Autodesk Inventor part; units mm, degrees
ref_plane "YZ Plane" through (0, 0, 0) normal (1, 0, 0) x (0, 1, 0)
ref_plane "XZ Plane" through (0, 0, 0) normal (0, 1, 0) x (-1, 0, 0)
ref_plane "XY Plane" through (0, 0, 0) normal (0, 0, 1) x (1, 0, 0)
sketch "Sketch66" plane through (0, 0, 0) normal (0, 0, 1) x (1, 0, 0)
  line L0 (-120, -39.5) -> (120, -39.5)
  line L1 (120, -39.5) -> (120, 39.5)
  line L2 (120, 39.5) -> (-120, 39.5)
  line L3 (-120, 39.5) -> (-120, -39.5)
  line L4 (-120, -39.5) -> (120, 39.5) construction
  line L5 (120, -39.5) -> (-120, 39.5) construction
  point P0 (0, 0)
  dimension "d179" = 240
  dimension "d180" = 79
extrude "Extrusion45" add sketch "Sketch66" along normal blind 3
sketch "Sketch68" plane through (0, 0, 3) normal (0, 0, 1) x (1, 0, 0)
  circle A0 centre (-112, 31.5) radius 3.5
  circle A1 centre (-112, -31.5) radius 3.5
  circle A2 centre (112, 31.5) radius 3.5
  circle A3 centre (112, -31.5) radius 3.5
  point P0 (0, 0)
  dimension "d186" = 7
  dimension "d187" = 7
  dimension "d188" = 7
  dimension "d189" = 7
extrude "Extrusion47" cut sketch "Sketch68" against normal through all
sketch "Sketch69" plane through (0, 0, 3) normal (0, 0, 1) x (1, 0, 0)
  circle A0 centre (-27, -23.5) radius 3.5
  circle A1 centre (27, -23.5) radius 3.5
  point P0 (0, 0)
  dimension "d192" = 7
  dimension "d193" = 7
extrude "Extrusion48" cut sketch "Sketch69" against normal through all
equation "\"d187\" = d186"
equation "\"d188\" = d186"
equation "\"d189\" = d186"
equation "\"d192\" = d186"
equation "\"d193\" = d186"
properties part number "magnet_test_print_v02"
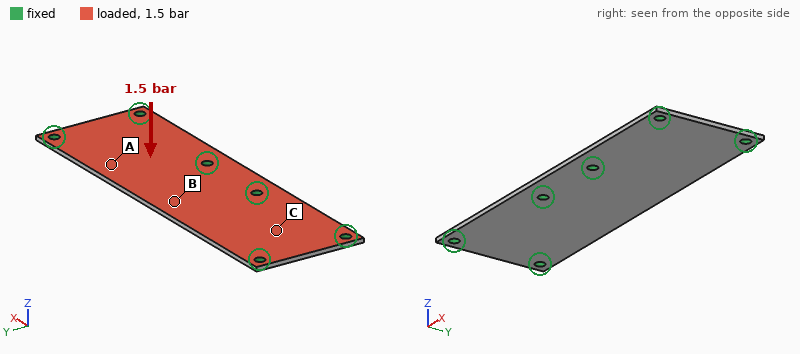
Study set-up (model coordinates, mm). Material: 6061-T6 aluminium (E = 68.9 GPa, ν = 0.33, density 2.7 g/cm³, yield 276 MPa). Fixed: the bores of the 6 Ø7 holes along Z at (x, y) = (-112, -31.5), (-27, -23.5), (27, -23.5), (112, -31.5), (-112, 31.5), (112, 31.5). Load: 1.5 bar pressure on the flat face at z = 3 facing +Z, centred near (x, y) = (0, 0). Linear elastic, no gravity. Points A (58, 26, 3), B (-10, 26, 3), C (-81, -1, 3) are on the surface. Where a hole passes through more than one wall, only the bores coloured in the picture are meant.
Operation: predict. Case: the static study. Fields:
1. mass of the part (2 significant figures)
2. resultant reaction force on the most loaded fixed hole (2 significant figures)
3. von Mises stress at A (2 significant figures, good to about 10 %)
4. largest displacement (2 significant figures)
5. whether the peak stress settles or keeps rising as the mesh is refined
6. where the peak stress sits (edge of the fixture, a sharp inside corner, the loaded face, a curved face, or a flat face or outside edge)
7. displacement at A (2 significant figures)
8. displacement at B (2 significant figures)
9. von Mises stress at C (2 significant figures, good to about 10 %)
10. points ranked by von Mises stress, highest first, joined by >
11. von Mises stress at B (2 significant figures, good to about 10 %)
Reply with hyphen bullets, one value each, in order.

- 150 g
- 770 N
- 61 MPa
- 1.4 mm
- keeps rising
- edge of the fixture
- 0.69 mm
- 0.99 mm
- 38 MPa
- A > C > B
- 20 MPa
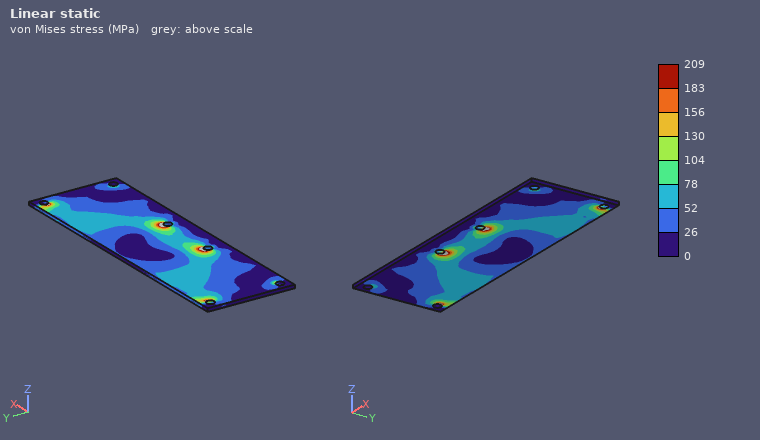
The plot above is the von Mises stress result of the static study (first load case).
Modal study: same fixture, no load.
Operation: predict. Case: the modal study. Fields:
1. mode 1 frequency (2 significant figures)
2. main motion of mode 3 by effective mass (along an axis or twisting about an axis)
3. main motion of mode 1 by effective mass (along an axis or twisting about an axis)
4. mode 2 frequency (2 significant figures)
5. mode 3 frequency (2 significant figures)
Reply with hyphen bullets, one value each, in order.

- 790 Hz
- along Z
- along Z
- 1300 Hz
- 1900 Hz
